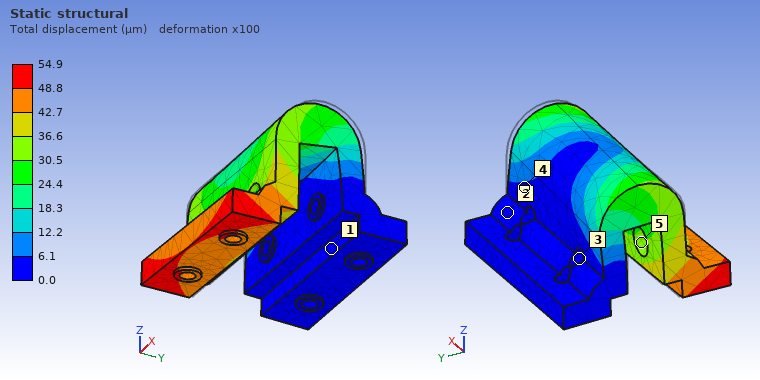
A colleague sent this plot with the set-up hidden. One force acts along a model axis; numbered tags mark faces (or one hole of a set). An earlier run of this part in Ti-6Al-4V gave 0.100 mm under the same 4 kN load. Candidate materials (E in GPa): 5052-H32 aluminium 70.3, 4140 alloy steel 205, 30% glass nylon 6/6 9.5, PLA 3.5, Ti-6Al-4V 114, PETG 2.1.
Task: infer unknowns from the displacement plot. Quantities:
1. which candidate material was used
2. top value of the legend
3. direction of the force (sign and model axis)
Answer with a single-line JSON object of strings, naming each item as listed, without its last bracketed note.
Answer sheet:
{"which candidate material was used": "4140 alloy steel", "top value of the legend": "54.9 µm", "direction of the force": "-X"}
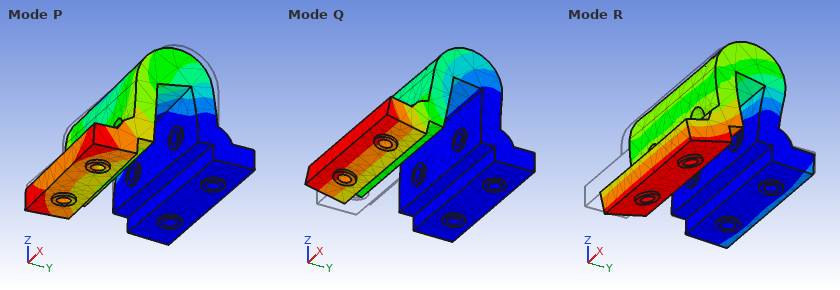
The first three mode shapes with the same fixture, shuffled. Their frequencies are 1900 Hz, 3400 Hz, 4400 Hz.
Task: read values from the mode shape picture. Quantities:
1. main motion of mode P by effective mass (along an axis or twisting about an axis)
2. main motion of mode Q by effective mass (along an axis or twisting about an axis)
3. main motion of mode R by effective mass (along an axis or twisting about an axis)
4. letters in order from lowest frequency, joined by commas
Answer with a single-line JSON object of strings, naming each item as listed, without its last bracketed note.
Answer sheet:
{"main motion of mode P by effective mass": "along X", "main motion of mode Q by effective mass": "along Z", "main motion of mode R by effective mass": "along Y", "letters in order from lowest frequency, joined by commas": "Q, P, R"}
